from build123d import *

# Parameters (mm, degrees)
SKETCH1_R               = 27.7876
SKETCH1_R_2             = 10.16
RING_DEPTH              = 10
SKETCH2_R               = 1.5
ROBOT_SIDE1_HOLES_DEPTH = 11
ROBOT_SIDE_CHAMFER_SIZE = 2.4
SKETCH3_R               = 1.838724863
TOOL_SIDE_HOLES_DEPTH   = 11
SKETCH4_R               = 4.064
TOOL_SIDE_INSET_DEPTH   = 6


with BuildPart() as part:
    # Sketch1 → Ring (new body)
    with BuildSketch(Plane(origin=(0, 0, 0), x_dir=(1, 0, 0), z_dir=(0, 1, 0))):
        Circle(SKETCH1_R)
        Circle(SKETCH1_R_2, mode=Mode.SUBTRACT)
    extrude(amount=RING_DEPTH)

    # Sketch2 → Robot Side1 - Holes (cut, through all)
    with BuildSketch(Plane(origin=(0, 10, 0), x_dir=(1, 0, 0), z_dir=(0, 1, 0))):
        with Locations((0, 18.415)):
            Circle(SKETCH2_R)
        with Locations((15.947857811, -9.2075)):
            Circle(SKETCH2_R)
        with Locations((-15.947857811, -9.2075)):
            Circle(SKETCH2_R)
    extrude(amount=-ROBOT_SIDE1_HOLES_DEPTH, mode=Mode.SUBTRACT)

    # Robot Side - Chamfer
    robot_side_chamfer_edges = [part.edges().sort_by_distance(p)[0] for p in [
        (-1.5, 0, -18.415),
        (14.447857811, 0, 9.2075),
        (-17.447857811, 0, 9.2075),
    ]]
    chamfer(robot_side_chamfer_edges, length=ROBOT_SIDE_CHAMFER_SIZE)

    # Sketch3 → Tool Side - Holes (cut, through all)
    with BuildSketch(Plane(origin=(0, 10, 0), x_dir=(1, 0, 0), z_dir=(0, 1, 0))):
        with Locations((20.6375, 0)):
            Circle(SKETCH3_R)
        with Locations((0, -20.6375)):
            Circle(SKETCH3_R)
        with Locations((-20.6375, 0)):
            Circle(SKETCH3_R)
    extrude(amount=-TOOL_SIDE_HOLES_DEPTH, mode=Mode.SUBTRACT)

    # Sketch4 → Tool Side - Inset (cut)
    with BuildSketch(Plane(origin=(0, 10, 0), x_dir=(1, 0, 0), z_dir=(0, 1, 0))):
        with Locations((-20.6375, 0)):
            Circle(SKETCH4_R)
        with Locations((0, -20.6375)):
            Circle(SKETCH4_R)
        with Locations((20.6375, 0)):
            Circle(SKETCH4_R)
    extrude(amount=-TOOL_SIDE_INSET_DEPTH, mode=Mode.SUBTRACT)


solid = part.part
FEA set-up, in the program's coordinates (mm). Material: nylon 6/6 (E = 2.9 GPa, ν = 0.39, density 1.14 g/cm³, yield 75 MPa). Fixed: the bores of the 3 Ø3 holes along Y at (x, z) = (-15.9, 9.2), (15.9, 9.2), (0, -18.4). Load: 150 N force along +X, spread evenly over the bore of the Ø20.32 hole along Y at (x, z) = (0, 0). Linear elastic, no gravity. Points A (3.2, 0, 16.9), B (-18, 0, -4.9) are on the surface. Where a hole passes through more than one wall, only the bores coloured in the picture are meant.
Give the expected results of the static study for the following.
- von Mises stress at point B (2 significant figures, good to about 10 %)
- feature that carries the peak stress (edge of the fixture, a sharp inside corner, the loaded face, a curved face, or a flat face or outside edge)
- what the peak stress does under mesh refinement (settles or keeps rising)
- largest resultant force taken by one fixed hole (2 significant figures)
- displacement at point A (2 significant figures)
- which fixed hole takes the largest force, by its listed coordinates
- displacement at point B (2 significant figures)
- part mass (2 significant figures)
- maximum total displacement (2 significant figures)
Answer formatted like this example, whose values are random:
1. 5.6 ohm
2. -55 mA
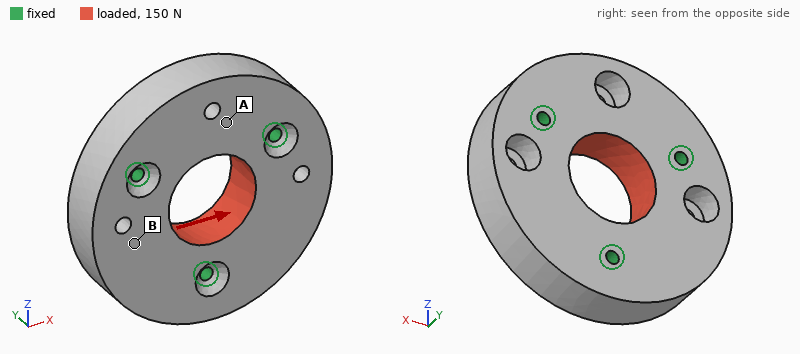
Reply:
1. 0.25 MPa
2. edge of the fixture
3. keeps rising
4. 56 N
5. 0.94 µm
6. (0, -18.4)
7. 2.6 µm
8. 22 g
9. 3.2 µm
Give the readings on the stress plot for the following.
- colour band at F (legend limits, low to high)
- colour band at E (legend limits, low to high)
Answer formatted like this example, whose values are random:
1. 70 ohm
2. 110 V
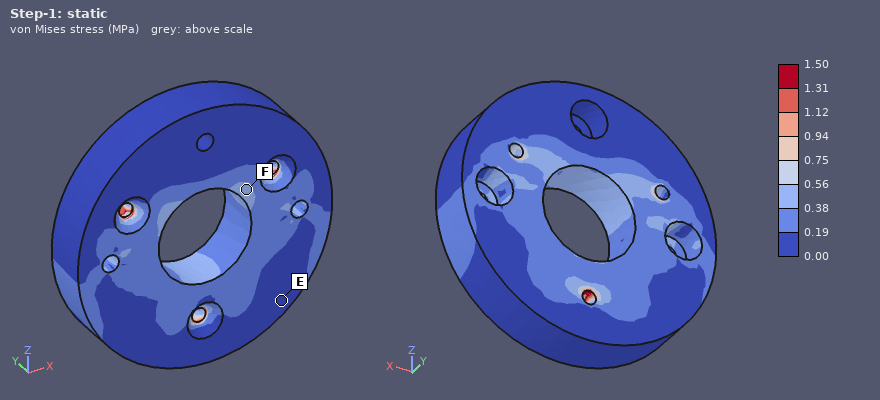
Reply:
1. 0.38 to 0.56 MPa
2. 0.00 to 0.19 MPa
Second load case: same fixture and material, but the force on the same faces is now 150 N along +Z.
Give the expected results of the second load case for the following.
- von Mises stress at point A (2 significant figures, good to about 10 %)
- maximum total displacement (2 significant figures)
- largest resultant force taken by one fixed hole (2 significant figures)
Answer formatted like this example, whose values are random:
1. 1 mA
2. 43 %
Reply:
1. 0.30 MPa
2. 3.8 µm
3. 52 N
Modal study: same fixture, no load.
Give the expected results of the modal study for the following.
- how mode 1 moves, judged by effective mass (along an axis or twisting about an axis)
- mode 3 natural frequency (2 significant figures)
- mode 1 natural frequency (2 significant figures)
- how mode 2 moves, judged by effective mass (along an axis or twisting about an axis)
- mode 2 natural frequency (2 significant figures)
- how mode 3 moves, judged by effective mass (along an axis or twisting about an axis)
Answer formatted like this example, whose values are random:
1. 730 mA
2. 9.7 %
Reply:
1. twisting about Z
2. 5700 Hz
3. 4200 Hz
4. twisting about X
5. 4400 Hz
6. along Y
